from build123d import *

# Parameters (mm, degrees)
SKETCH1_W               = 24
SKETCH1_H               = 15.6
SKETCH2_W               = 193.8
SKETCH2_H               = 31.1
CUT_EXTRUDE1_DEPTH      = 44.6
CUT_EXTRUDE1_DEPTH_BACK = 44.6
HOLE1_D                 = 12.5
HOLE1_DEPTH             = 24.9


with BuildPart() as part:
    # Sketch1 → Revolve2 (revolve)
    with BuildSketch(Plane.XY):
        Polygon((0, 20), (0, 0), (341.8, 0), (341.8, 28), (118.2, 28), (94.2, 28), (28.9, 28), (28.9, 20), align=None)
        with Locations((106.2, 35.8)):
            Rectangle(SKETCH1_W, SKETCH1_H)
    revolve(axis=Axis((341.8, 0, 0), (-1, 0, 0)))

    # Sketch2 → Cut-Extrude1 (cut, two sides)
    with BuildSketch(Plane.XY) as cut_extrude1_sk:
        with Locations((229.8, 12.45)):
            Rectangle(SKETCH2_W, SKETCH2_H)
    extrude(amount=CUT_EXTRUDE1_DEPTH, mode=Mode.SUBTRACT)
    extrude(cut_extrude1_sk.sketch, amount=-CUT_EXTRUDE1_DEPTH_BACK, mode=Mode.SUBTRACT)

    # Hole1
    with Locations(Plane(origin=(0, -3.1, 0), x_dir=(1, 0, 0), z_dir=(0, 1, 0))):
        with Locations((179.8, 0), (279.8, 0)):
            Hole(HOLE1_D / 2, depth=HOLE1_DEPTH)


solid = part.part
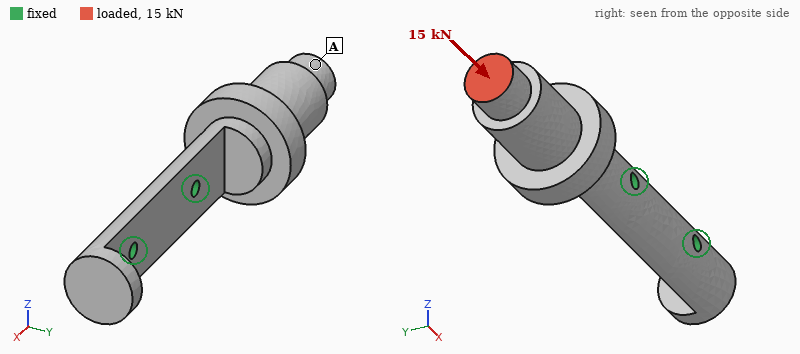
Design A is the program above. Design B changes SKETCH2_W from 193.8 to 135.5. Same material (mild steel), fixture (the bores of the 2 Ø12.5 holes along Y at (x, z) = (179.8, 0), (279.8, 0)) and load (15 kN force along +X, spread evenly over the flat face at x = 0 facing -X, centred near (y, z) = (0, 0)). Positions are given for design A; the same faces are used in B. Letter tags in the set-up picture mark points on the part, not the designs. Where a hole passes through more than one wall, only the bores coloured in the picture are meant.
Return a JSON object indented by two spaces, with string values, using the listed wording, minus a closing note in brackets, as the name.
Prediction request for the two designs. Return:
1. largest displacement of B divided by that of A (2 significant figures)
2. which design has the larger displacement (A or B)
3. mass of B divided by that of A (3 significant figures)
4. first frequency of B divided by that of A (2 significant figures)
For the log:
{
  "largest displacement of B divided by that of A": "0.54",
  "which design has the larger displacement": "A",
  "mass of B divided by that of A": "1.13",
  "first frequency of B divided by that of A": "1.2"
}
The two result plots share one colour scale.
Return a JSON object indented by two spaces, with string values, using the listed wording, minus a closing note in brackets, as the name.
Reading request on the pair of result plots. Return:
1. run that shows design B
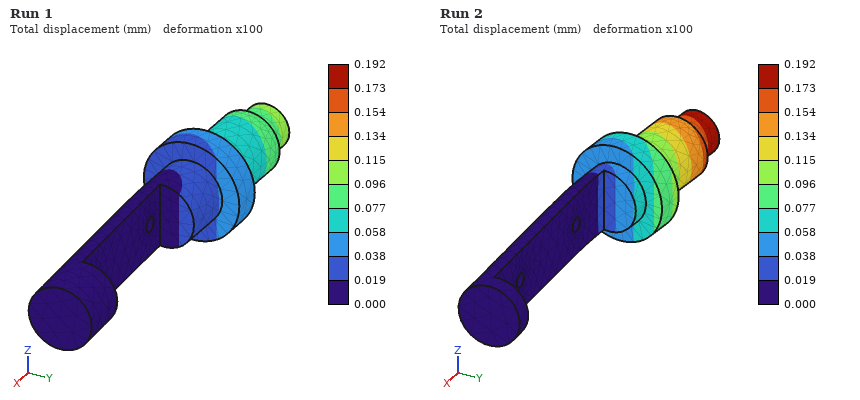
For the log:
{
  "run that shows design B": "Run 1"
}
